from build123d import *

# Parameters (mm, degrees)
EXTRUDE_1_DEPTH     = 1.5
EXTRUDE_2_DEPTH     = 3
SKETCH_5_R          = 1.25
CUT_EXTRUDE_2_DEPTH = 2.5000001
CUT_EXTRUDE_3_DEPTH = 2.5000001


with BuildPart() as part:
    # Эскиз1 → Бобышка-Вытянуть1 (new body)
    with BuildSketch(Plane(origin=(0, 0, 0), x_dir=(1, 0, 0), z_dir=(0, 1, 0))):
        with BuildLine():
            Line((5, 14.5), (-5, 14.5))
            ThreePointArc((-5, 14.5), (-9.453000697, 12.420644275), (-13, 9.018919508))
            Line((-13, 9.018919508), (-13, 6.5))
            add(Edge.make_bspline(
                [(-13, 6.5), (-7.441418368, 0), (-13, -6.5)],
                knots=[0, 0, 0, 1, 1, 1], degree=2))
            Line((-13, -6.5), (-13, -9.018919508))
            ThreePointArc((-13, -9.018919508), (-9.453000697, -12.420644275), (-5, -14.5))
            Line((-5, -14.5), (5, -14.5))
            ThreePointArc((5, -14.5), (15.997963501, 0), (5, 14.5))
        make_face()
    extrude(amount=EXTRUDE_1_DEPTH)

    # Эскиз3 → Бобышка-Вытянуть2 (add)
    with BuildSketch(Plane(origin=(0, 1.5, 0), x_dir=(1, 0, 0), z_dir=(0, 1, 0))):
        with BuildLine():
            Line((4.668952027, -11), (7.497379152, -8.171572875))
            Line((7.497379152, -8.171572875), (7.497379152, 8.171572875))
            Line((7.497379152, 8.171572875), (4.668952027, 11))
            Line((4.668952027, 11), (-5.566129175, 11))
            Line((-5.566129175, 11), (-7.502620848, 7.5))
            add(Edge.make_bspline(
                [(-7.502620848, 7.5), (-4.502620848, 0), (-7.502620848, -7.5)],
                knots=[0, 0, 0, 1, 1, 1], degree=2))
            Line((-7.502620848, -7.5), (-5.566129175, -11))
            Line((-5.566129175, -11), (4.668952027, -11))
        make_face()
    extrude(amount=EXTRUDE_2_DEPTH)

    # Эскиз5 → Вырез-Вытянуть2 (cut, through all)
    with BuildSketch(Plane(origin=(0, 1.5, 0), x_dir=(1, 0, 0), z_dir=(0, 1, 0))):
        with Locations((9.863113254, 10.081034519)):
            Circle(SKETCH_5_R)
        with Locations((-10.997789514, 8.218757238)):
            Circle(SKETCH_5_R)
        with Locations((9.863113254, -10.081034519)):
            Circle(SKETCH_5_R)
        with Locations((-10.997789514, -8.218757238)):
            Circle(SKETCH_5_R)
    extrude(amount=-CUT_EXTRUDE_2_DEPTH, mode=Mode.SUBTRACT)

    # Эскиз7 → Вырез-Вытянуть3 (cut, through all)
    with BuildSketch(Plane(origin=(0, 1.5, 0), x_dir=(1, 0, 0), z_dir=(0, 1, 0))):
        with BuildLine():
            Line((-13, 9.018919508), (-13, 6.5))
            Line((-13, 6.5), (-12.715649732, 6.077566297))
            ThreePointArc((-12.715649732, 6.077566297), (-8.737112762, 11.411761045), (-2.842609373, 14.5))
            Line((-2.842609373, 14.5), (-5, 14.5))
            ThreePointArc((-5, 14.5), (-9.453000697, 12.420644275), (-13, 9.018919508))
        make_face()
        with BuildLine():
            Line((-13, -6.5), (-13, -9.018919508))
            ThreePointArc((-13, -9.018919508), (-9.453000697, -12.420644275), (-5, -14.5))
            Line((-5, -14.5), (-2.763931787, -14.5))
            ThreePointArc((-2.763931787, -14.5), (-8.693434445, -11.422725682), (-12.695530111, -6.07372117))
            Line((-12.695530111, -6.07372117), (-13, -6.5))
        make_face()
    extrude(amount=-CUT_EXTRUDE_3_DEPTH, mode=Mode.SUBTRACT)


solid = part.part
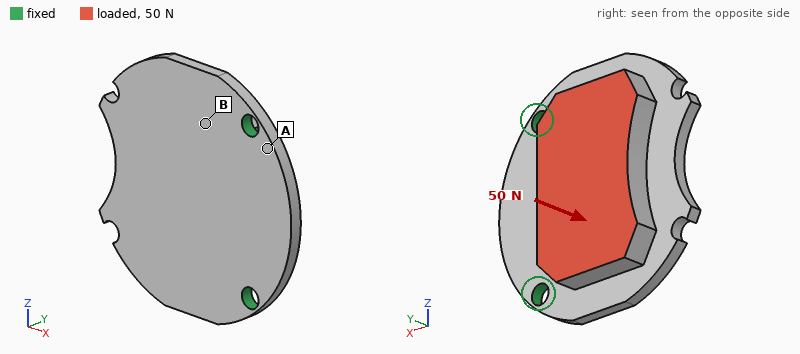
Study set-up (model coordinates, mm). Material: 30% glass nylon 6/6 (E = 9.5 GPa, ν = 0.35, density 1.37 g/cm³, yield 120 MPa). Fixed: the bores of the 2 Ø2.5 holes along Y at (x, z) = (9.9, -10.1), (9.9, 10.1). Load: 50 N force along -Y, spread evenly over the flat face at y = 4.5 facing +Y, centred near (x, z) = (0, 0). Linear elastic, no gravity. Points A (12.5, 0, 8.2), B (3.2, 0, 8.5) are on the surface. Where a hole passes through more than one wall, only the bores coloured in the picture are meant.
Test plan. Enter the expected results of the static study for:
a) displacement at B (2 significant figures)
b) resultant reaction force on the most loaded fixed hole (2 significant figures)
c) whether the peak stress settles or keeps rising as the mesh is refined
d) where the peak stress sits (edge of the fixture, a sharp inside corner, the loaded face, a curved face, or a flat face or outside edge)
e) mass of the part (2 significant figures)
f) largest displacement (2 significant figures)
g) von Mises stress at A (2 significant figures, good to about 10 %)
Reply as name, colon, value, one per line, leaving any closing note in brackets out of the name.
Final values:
displacement at B: 0.10 mm
resultant reaction force on the most loaded fixed hole: 27 N
whether the peak stress settles or keeps rising as the mesh is refined: keeps rising
where the peak stress sits: edge of the fixture
mass of the part: 2.6 g
largest displacement: 0.44 mm
von Mises stress at A: 14 MPa
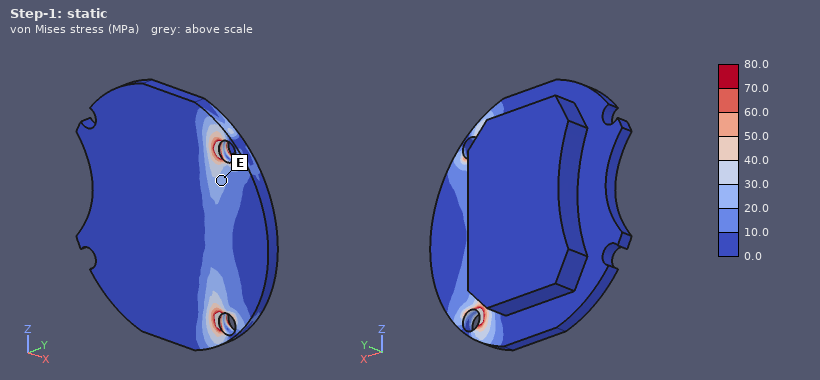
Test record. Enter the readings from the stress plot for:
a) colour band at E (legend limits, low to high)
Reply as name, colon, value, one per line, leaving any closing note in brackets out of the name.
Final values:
colour band at E: 20.0 to 30.0 MPa
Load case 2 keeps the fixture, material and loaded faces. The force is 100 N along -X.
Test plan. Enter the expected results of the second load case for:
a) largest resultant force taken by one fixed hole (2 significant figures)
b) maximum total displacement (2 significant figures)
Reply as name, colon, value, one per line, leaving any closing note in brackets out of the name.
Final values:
largest resultant force taken by one fixed hole: 50 N
maximum total displacement: 0.42 mm
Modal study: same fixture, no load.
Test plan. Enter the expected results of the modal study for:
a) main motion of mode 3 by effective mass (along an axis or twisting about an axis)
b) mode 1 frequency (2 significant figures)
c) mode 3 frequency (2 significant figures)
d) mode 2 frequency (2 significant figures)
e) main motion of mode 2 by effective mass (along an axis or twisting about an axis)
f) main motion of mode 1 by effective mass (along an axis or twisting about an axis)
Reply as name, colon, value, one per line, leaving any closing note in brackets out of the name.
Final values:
main motion of mode 3 by effective mass: along Y
mode 1 frequency: 1500 Hz
mode 3 frequency: 11 kHz
mode 2 frequency: 6800 Hz
main motion of mode 2 by effective mass: twisting about X
main motion of mode 1 by effective mass: along Y
